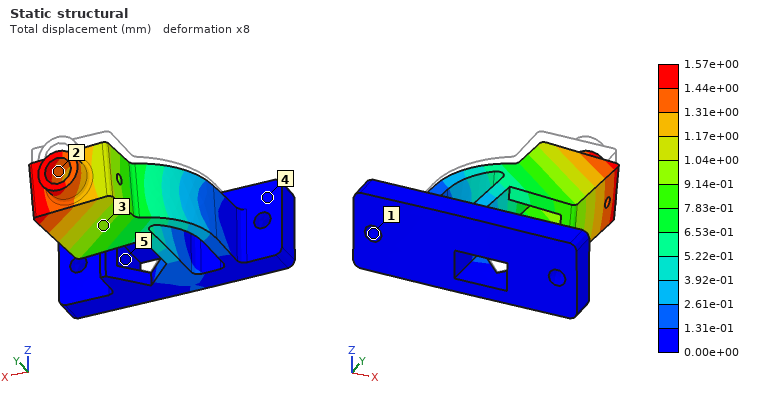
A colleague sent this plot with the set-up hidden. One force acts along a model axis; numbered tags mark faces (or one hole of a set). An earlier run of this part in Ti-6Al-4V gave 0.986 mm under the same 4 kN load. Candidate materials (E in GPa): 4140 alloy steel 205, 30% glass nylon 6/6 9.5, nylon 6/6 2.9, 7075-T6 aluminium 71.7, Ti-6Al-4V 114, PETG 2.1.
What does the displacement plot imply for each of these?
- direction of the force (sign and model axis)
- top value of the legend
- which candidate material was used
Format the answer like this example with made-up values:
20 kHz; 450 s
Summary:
-Z; 1.57e+00 mm; 7075-T6 aluminium
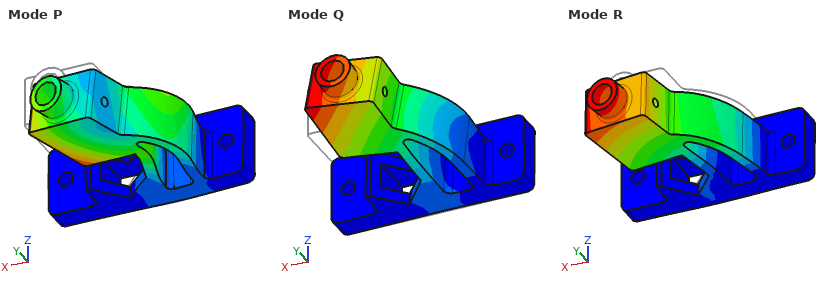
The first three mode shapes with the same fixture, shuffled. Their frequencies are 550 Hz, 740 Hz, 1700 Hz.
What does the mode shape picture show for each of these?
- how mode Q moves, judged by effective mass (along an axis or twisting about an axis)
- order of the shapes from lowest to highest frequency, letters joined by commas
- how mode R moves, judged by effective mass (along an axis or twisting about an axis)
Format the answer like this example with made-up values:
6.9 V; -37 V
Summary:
along Z; Q, R, P; along X
